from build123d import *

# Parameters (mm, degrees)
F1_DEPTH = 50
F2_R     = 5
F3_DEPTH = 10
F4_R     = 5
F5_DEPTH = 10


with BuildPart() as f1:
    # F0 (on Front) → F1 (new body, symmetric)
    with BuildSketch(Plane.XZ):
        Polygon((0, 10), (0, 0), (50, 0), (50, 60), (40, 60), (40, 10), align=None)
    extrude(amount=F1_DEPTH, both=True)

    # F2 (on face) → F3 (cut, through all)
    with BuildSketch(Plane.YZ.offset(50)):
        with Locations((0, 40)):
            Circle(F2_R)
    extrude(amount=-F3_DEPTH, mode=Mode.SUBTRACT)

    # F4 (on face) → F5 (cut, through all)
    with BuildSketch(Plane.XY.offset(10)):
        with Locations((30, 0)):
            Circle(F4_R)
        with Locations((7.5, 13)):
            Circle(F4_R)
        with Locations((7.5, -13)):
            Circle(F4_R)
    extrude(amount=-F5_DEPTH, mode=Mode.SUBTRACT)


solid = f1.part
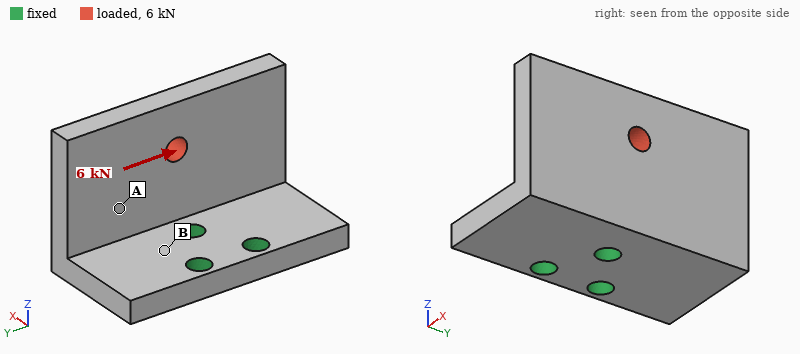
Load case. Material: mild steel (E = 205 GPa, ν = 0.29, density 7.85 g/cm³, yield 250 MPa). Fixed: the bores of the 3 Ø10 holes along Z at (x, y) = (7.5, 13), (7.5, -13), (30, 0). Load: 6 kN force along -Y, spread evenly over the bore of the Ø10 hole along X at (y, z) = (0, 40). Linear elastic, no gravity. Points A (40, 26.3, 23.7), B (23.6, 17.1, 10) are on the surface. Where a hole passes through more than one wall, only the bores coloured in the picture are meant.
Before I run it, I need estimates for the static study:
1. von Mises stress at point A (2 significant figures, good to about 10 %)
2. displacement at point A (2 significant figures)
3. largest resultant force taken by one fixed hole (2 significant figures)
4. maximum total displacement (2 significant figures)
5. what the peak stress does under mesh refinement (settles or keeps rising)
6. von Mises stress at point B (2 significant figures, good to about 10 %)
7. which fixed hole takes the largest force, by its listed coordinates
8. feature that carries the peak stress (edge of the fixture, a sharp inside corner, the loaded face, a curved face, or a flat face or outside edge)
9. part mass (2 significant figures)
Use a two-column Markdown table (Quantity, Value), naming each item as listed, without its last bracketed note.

| Quantity | Value |
|---|---|
| von Mises stress at point A | 31 MPa |
| displacement at point A | 0.043 mm |
| largest resultant force taken by one fixed hole | 6.7 kN |
| maximum total displacement | 0.10 mm |
| what the peak stress does under mesh refinement | keeps rising |
| von Mises stress at point B | 62 MPa |
| which fixed hole takes the largest force, by its listed coordinates | (30, 0) |
| feature that carries the peak stress | edge of the fixture |
| part mass | 760 g |
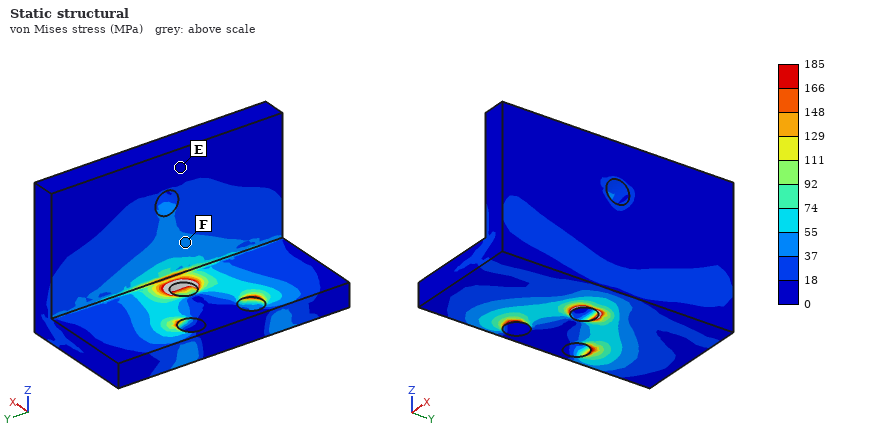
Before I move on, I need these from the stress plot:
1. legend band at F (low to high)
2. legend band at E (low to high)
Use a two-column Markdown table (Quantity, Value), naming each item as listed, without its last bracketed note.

| Quantity | Value |
|---|---|
| legend band at F | 37 to 55 MPa |
| legend band at E | 0 to 18 MPa |
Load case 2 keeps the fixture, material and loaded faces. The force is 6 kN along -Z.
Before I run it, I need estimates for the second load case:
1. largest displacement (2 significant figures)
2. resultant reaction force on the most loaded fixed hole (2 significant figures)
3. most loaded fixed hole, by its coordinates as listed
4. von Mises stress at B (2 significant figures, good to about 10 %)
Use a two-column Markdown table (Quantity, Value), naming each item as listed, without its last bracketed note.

| Quantity | Value |
|---|---|
| largest displacement | 36 µm |
| resultant reaction force on the most loaded fixed hole | 6.8 kN |
| most loaded fixed hole, by its coordinates as listed | (30, 0) |
| von Mises stress at B | 21 MPa |
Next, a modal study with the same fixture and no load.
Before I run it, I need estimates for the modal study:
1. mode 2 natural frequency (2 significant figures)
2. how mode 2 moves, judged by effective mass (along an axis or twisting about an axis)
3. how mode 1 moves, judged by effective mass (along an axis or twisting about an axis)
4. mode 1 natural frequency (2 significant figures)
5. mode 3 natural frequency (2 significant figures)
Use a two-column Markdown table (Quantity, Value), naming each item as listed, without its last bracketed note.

| Quantity | Value |
|---|---|
| mode 2 natural frequency | 2100 Hz |
| how mode 2 moves, judged by effective mass | along Y |
| how mode 1 moves, judged by effective mass | along X |
| mode 1 natural frequency | 1900 Hz |
| mode 3 natural frequency | 3600 Hz |
